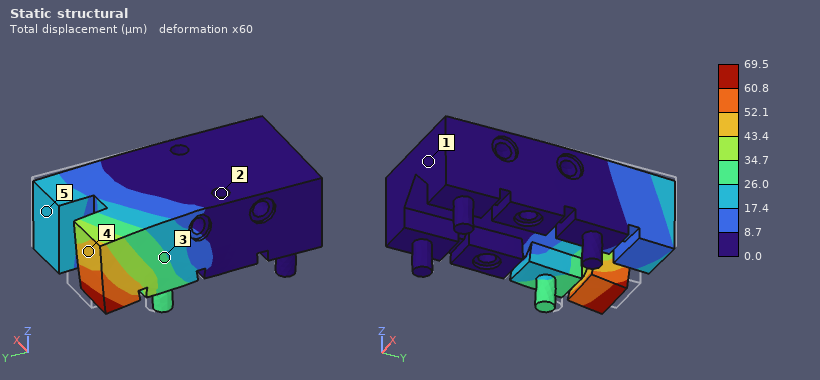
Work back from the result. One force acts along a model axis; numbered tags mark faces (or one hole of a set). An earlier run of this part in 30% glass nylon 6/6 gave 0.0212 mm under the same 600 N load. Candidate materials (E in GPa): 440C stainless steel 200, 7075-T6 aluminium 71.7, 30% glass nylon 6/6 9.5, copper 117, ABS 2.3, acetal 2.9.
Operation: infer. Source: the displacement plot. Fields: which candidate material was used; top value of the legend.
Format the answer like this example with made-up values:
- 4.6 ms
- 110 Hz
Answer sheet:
- acetal
- 69.5 µm
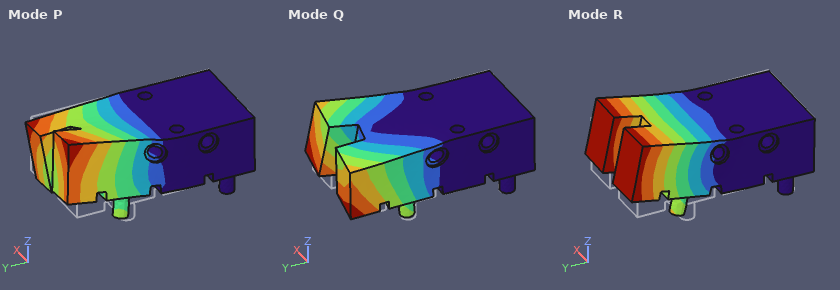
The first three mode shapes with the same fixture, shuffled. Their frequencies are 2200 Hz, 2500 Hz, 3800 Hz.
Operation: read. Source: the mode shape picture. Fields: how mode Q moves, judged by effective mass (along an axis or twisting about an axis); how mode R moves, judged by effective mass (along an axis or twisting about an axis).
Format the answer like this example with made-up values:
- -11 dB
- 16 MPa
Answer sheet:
- along X
- along Z
